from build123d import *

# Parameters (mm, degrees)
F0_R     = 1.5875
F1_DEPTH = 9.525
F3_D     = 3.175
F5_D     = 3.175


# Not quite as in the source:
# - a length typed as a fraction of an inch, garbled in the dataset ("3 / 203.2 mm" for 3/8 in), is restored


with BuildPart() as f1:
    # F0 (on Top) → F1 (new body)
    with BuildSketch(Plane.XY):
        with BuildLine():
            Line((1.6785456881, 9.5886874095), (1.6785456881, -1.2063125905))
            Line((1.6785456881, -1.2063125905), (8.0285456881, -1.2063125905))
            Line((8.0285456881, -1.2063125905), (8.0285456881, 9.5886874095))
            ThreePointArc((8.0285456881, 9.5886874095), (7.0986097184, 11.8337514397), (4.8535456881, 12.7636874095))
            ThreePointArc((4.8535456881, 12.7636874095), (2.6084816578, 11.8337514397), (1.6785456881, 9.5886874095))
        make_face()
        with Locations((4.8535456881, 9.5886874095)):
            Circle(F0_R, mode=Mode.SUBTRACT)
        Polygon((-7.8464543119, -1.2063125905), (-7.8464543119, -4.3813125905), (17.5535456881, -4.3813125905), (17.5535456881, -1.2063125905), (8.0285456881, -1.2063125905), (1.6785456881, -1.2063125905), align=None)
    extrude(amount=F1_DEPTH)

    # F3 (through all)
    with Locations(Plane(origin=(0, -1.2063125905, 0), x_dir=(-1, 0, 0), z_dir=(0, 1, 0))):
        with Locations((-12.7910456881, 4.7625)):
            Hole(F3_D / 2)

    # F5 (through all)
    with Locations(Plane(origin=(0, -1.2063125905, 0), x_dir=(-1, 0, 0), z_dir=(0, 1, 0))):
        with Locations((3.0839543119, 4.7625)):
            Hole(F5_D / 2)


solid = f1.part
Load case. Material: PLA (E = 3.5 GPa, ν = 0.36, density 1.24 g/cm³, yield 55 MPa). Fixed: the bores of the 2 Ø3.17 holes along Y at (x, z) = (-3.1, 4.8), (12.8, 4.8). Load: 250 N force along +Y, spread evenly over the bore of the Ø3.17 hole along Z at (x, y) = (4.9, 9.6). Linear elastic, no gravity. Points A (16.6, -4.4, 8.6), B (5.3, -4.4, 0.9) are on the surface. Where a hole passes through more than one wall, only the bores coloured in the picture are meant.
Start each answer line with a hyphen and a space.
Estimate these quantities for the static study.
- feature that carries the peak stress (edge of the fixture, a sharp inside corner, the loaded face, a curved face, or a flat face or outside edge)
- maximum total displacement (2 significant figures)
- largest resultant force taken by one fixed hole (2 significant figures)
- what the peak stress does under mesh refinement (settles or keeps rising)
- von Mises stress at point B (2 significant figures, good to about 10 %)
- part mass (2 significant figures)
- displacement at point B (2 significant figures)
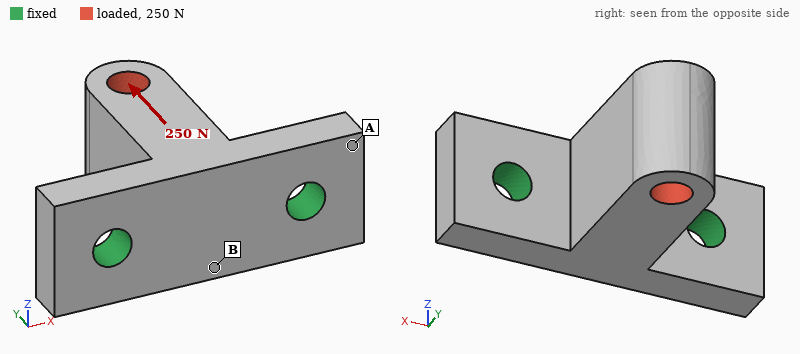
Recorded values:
- edge of the fixture
- 59 µm
- 130 N
- keeps rising
- 8.6 MPa
- 1.8 g
- 40 µm
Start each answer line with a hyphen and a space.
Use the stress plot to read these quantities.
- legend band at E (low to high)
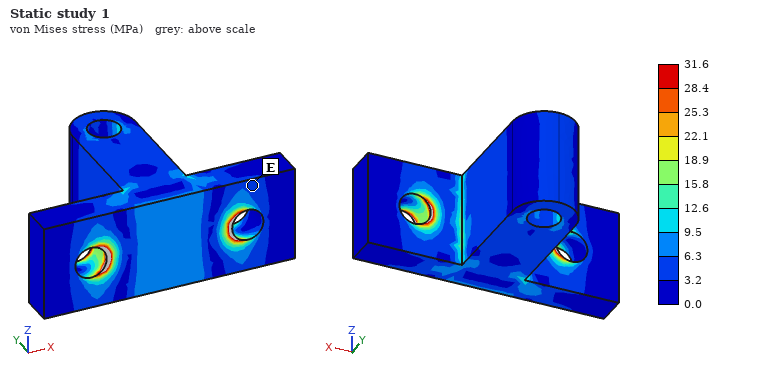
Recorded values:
- 3.2 to 6.3 MPa
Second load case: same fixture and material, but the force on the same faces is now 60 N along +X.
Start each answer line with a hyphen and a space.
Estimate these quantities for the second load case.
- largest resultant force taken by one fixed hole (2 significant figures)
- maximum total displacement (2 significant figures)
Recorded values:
- 73 N
- 0.13 mm
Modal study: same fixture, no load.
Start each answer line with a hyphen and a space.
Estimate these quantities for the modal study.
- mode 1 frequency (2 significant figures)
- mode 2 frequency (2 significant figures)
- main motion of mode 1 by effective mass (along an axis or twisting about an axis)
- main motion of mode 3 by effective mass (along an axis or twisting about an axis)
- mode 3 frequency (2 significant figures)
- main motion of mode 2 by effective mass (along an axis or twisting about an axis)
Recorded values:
- 4000 Hz
- 6100 Hz
- along Z
- along Y
- 11 kHz
- along X
